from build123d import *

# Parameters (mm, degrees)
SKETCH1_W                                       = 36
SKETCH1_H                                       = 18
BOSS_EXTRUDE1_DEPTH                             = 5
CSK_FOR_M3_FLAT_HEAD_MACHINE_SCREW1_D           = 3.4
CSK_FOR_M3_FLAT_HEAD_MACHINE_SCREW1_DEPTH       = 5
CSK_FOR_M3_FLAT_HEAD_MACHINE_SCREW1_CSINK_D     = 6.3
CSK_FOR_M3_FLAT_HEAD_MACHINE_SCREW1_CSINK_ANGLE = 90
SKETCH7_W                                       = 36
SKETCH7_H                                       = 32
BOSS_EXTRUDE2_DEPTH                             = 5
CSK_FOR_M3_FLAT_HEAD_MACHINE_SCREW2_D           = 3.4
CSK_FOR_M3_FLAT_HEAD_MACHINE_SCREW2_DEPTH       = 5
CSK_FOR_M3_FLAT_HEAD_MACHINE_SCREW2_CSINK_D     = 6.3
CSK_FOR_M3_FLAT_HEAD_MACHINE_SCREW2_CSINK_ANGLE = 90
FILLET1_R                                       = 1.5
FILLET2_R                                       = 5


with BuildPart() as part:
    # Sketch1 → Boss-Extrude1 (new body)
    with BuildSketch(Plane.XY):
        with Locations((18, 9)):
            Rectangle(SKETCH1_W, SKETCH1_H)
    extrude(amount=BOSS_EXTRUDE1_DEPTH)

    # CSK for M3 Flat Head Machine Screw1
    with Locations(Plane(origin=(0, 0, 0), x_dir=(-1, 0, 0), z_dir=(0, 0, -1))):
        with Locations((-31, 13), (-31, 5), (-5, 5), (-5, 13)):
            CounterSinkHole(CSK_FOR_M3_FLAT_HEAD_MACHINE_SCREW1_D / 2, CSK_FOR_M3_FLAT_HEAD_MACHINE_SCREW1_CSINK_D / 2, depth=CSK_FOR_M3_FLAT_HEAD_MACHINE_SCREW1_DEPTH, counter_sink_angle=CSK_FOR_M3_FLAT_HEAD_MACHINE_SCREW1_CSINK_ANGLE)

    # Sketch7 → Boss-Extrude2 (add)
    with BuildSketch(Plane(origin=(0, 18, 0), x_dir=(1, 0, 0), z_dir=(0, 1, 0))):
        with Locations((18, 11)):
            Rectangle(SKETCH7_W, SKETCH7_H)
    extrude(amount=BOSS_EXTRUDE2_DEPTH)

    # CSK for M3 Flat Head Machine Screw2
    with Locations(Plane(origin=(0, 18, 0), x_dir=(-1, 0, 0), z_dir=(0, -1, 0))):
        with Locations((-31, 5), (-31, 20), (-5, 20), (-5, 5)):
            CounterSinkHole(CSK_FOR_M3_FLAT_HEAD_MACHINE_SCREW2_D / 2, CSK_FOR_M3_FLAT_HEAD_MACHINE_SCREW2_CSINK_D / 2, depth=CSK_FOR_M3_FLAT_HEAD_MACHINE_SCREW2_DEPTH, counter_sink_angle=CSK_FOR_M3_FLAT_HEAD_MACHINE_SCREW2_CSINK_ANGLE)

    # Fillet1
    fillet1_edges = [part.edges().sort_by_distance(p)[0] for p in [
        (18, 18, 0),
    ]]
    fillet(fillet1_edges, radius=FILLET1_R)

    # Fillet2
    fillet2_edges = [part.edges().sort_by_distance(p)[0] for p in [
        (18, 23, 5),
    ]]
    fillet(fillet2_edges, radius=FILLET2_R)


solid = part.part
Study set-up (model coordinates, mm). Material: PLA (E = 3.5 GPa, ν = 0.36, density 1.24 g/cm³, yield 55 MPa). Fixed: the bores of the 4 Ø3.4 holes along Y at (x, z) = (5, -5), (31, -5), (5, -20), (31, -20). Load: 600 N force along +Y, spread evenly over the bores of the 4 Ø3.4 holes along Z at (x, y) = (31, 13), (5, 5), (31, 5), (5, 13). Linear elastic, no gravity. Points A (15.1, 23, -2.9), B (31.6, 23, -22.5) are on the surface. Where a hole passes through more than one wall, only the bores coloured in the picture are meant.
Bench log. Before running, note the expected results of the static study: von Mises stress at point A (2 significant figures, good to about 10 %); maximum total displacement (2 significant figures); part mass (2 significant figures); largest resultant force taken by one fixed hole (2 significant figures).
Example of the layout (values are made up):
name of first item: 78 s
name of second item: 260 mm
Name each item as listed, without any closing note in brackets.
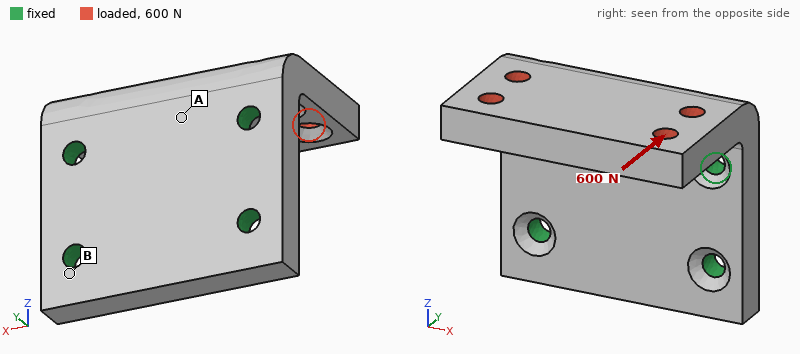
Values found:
von Mises stress at point A: 12 MPa
maximum total displacement: 0.56 mm
part mass: 10 g
largest resultant force taken by one fixed hole: 370 N
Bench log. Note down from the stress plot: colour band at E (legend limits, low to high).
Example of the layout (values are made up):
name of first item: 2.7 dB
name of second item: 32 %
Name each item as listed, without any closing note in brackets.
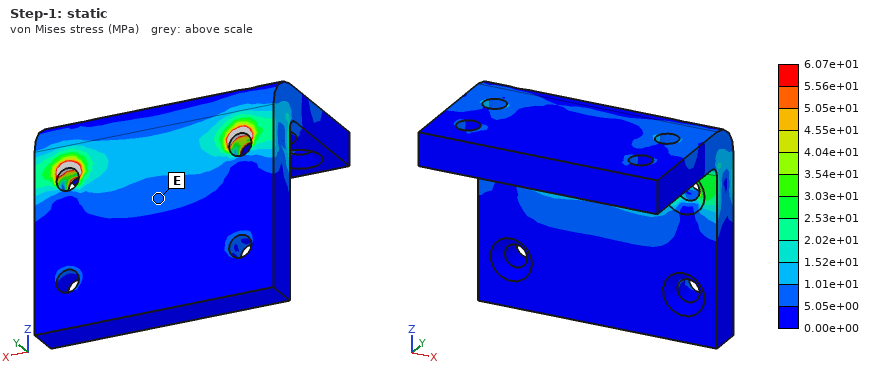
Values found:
colour band at E: 5.05e+00 to 1.01e+01 MPa
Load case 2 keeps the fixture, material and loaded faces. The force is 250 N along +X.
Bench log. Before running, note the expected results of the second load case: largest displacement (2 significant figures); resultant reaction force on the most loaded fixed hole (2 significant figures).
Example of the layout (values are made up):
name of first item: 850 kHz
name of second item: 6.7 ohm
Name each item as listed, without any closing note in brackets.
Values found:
largest displacement: 91 µm
resultant reaction force on the most loaded fixed hole: 180 N
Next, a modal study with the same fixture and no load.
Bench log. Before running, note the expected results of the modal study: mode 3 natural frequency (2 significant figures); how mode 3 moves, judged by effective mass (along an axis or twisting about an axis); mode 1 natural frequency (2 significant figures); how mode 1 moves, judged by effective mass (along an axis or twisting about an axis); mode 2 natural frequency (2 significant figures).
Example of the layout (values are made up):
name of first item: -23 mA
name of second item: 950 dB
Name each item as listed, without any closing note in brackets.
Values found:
mode 3 natural frequency: 5800 Hz
how mode 3 moves, judged by effective mass: along X
mode 1 natural frequency: 2000 Hz
how mode 1 moves, judged by effective mass: along Z
mode 2 natural frequency: 3700 Hz
